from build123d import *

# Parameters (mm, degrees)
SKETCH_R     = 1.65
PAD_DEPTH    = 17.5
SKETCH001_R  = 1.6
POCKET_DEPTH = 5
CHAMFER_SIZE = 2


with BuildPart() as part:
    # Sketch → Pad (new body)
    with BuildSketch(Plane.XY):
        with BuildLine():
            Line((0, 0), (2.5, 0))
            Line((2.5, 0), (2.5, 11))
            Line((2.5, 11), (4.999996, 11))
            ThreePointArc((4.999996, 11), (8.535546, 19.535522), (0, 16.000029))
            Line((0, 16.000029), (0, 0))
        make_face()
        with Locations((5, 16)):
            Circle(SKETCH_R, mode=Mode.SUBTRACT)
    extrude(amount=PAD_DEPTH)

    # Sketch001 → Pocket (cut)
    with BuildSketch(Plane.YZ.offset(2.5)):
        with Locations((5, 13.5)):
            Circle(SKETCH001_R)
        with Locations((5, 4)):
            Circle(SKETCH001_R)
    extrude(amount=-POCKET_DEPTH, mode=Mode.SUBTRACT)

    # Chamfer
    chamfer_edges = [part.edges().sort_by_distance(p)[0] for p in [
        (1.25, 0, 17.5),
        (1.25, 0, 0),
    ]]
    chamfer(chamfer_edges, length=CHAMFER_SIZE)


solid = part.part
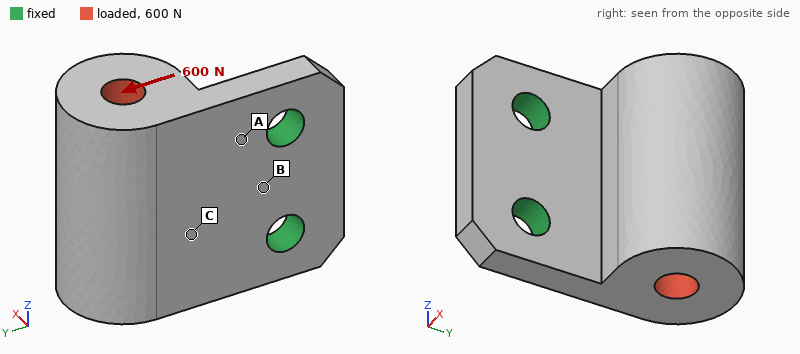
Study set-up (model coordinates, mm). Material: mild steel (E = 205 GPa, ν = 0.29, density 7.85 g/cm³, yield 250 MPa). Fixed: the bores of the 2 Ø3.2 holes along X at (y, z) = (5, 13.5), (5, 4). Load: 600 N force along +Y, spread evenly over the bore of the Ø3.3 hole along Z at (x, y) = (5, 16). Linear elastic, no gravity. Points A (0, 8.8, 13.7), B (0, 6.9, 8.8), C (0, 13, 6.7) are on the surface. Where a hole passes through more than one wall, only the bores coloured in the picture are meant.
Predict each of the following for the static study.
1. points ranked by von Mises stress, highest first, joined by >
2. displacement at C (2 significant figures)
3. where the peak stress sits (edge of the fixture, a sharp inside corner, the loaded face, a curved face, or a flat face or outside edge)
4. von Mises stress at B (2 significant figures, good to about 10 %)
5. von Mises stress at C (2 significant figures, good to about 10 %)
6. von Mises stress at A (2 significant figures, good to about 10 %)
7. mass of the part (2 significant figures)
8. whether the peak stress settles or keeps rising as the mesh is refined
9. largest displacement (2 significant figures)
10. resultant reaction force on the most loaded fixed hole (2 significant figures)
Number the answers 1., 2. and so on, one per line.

1. A > B > C
2. 12 µm
3. edge of the fixture
4. 70 MPa
5. 30 MPa
6. 100 MPa
7. 14 g
8. keeps rising
9. 39 µm
10. 300 N
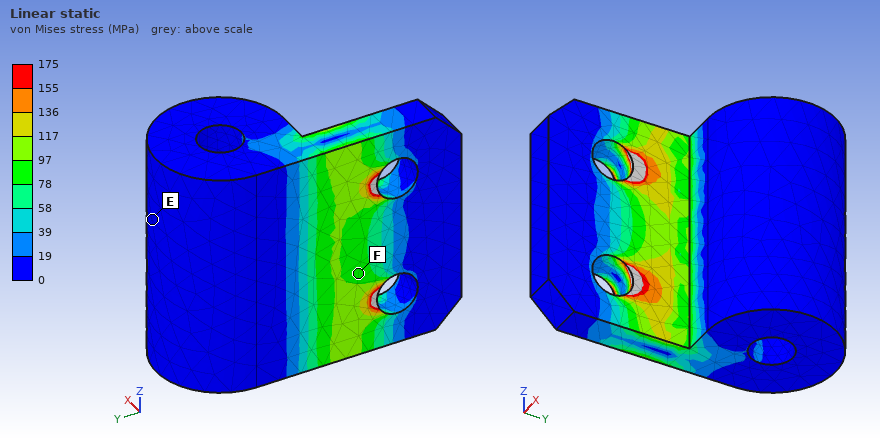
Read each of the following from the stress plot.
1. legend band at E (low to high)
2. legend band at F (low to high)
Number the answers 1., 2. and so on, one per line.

1. 0 to 19 MPa
2. 78 to 97 MPa
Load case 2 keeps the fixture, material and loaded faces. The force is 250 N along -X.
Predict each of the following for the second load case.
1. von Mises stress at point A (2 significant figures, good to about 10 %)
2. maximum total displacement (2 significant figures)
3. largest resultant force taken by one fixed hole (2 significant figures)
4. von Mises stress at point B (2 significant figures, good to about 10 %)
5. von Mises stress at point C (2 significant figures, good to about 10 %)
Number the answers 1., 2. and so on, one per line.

1. 99 MPa
2. 32 µm
3. 130 N
4. 73 MPa
5. 21 MPa
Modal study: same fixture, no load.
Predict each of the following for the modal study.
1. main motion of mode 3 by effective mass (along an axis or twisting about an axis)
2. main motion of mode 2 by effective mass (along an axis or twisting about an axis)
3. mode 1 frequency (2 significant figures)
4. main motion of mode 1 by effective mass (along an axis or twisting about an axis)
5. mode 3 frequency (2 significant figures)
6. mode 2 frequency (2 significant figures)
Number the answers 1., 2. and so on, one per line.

1. along Z
2. along Z
3. 4900 Hz
4. along X
5. 24 kHz
6. 14 kHz
